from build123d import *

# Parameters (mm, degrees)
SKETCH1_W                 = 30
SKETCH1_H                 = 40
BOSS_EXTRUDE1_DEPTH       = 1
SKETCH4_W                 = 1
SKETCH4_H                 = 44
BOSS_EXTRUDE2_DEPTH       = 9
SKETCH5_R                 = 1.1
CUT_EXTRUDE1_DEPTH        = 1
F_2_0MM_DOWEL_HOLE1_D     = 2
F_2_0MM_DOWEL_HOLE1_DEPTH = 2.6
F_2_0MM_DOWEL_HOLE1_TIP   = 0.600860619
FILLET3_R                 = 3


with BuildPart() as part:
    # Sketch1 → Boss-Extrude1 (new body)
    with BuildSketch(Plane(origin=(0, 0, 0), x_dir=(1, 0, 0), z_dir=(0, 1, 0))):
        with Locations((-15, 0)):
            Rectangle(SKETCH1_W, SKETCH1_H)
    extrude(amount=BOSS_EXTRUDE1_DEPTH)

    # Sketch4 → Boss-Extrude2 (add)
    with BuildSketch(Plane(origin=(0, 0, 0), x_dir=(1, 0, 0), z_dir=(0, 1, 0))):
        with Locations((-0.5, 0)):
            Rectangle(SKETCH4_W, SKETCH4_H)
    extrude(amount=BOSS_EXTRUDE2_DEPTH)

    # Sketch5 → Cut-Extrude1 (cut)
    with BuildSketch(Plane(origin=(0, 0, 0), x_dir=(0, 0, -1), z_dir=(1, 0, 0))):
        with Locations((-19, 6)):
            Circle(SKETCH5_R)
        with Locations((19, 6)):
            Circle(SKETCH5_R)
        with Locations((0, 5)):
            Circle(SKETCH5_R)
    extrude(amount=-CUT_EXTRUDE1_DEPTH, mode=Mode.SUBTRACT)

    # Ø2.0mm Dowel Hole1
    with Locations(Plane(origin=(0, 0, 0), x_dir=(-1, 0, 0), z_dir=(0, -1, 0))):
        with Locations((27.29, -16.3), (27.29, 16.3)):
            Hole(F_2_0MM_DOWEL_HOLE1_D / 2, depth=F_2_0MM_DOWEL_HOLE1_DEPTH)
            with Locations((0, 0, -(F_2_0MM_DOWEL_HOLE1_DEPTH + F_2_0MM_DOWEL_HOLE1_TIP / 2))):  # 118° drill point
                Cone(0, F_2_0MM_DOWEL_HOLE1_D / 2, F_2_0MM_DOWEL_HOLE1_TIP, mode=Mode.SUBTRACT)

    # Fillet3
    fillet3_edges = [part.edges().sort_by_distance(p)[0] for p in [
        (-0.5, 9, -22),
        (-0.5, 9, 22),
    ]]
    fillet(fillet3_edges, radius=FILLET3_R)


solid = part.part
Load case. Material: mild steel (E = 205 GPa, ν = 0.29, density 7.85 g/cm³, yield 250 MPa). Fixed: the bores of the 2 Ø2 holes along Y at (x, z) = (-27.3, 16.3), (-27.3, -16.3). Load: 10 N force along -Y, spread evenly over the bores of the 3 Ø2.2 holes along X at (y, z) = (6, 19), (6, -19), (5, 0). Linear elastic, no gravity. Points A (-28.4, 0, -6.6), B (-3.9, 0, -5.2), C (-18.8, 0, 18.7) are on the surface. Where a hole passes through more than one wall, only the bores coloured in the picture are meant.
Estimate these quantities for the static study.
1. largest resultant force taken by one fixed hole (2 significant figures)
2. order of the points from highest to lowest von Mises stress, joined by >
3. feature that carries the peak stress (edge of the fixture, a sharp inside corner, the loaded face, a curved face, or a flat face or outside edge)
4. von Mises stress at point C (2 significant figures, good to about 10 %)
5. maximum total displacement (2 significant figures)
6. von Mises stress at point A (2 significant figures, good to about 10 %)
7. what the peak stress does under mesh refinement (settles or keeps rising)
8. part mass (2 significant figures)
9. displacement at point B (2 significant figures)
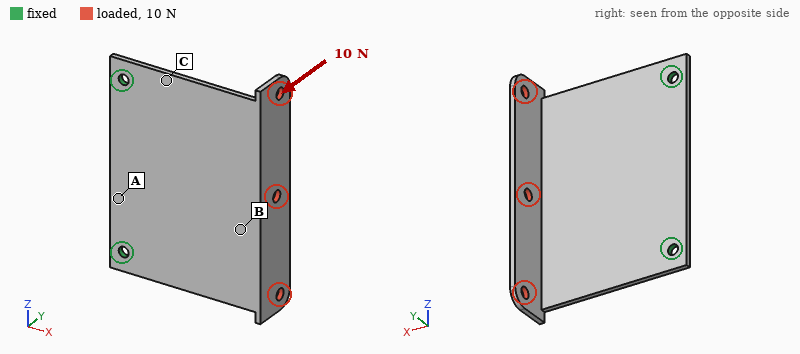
5.0 N
C > A > B
edge of the fixture
36 MPa
0.14 mm
20 MPa
keeps rising
12 g
0.11 mm
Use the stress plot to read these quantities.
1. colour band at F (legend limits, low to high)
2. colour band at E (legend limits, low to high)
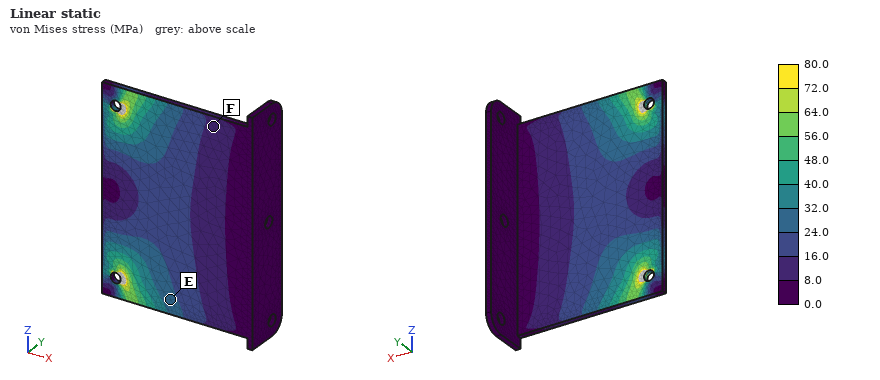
8.0 to 16.0 MPa
24.0 to 32.0 MPa
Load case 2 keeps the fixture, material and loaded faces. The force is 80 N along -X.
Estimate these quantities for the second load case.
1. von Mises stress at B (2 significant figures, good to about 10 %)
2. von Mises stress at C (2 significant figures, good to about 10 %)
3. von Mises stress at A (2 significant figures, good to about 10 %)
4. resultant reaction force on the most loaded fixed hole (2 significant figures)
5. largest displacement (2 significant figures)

51 MPa
73 MPa
37 MPa
41 N
0.33 mm
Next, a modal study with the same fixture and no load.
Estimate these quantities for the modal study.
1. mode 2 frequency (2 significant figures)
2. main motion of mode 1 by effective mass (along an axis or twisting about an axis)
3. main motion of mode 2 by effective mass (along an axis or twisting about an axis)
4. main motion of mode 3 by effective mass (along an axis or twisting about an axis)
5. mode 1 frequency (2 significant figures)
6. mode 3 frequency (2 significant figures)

1500 Hz
along Y
twisting about X
along Y
620 Hz
3700 Hz
